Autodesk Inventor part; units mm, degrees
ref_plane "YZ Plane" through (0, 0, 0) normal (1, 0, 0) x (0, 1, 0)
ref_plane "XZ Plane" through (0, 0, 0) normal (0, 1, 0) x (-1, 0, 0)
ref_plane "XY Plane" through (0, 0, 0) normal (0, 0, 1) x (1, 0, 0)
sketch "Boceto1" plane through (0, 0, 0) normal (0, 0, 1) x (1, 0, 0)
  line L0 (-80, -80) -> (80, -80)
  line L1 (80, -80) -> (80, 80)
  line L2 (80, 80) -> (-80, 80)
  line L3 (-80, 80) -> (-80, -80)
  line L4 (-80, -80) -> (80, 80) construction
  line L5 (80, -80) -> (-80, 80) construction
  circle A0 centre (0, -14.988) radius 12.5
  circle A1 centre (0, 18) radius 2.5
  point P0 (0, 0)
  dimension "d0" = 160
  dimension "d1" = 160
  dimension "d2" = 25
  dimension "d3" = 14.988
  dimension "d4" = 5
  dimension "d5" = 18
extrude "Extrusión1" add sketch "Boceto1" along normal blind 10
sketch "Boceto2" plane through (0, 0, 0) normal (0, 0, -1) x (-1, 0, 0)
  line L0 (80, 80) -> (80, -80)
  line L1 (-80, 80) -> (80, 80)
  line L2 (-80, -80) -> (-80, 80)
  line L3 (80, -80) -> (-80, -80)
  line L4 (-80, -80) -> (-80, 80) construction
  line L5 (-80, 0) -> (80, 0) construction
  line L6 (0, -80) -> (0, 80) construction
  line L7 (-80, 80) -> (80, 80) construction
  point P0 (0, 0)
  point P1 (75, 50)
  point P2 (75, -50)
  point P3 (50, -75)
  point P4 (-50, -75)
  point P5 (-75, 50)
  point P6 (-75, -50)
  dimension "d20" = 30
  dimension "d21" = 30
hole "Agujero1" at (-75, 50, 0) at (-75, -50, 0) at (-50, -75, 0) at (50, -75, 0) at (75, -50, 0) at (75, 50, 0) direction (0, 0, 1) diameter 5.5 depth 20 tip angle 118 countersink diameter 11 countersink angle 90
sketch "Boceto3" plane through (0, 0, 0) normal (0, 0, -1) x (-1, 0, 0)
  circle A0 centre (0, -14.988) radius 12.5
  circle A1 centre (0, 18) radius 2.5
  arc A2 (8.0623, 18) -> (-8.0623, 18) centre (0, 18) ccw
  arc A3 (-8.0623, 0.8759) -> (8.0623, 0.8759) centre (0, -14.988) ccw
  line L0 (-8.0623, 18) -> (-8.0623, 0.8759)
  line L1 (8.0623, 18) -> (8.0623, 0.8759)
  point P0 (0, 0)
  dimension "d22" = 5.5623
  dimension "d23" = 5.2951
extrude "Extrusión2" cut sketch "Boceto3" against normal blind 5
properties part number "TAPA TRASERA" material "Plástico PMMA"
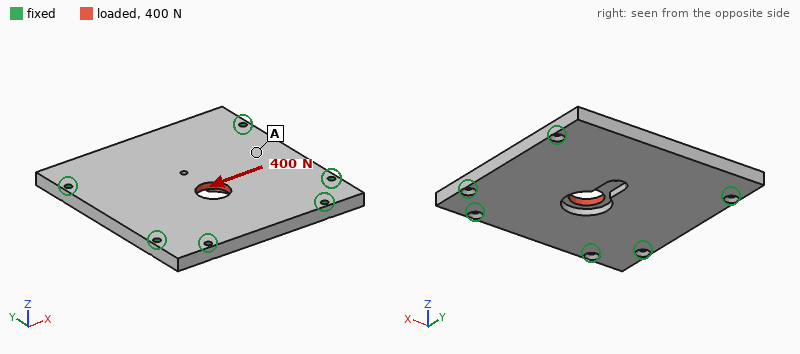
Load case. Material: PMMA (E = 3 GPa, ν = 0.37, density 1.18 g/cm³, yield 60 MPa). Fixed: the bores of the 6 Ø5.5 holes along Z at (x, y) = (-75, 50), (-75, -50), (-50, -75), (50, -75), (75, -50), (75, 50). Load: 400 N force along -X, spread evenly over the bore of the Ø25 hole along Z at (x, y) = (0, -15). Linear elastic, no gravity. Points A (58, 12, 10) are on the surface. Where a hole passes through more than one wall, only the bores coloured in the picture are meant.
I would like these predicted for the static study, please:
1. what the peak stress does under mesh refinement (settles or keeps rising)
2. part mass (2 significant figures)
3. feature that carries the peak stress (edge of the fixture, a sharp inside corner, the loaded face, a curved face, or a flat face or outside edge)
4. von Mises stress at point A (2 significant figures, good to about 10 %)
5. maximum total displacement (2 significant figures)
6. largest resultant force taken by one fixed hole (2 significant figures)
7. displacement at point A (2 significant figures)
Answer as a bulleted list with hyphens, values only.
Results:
- keeps rising
- 290 g
- edge of the fixture
- 0.18 MPa
- 15 µm
- 82 N
- 7.2 µm
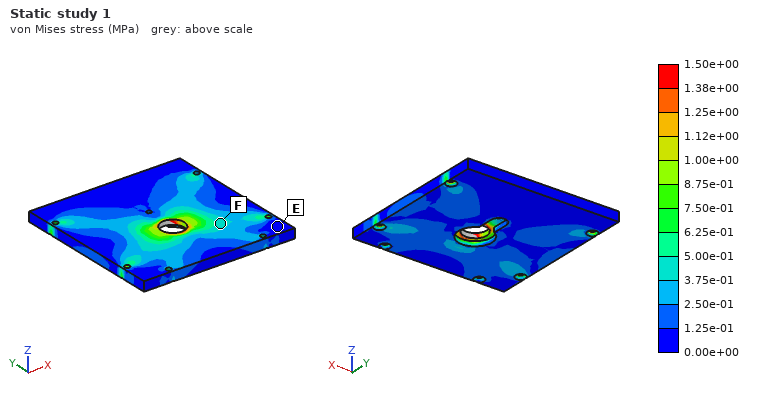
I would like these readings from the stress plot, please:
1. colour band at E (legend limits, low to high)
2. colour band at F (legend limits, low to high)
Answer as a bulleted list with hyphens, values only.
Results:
- 0.00e+00 to 1.25e-01 MPa
- 3.75e-01 to 5.00e-01 MPa
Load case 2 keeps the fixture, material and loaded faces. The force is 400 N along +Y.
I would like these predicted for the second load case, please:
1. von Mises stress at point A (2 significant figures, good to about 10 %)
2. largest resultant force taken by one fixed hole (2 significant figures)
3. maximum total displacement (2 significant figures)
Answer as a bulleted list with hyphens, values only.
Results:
- 0.22 MPa
- 98 N
- 17 µm
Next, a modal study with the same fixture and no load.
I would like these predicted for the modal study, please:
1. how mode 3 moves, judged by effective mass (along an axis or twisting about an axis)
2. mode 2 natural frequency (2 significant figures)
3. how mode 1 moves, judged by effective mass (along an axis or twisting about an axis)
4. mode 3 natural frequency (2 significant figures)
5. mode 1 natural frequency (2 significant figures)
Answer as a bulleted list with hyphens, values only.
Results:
- twisting about Y
- 780 Hz
- along Z
- 1200 Hz
- 520 Hz
